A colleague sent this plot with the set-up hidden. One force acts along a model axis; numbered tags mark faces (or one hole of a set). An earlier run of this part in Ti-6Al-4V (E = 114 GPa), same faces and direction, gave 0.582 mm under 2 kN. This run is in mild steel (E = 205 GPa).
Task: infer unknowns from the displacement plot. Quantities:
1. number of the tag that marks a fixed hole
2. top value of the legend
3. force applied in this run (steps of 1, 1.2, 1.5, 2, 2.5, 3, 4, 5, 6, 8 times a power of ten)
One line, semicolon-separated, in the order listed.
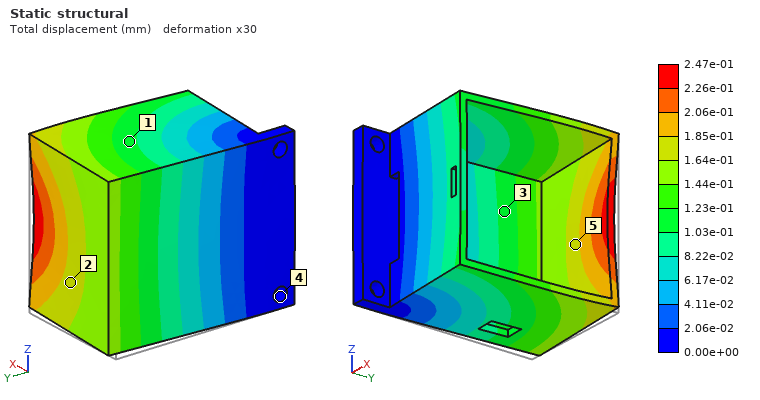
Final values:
4; 2.47e-01 mm; 1.5 kN
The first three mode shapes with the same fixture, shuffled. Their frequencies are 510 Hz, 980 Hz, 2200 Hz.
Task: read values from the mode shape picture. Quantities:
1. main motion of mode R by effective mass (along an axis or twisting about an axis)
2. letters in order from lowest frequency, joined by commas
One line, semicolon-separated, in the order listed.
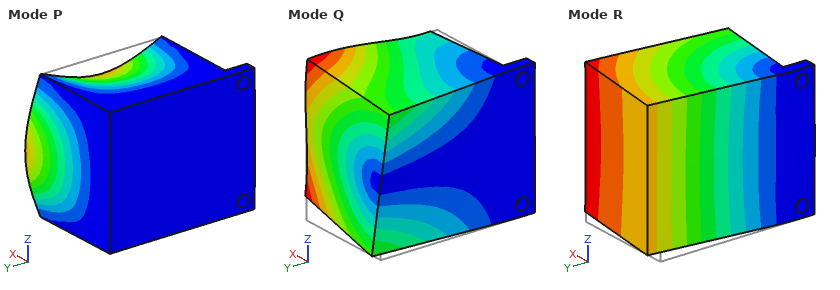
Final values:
along X; R, Q, P
